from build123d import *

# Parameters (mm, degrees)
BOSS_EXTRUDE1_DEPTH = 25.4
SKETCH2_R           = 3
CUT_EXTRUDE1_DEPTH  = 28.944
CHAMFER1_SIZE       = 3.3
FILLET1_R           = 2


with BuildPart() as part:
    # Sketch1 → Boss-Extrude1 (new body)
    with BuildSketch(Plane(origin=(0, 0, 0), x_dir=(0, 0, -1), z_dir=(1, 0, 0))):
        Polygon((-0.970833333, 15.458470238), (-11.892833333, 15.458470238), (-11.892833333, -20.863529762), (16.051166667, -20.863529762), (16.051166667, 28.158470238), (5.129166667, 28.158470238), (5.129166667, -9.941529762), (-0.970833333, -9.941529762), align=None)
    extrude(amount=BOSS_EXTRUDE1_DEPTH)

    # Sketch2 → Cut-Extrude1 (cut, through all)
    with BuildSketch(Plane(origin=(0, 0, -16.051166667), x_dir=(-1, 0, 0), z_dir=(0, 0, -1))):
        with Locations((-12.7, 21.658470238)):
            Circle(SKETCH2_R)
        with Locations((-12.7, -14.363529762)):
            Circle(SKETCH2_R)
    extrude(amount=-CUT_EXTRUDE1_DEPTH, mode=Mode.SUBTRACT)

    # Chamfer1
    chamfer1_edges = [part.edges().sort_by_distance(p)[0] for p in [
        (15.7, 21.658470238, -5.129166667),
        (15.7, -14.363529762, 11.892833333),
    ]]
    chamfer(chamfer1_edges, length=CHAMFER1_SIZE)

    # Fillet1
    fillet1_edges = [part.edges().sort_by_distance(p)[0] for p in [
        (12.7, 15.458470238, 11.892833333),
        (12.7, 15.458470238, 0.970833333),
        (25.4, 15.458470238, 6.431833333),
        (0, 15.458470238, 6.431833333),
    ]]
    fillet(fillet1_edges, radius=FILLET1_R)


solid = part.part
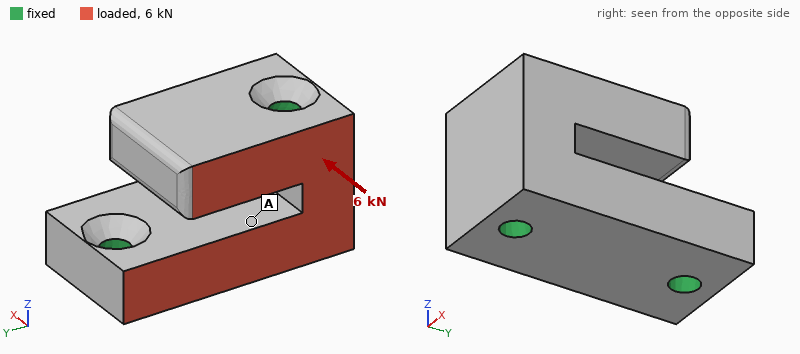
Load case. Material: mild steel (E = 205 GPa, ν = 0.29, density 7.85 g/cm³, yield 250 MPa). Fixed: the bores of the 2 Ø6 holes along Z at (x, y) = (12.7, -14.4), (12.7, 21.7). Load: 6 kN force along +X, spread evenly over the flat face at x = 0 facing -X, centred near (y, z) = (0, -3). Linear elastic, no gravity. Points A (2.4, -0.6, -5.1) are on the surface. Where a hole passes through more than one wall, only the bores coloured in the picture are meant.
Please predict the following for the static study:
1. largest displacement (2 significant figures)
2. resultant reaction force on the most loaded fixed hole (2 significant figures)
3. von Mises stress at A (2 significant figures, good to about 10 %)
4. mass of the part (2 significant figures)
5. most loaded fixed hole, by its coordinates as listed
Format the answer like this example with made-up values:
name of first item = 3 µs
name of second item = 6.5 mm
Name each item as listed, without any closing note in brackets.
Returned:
largest displacement = 8.3 µm
resultant reaction force on the most loaded fixed hole = 4.3 kN
von Mises stress at A = 7.4 MPa
mass of the part = 190 g
most loaded fixed hole, by its coordinates as listed = (12.7, -14.4)
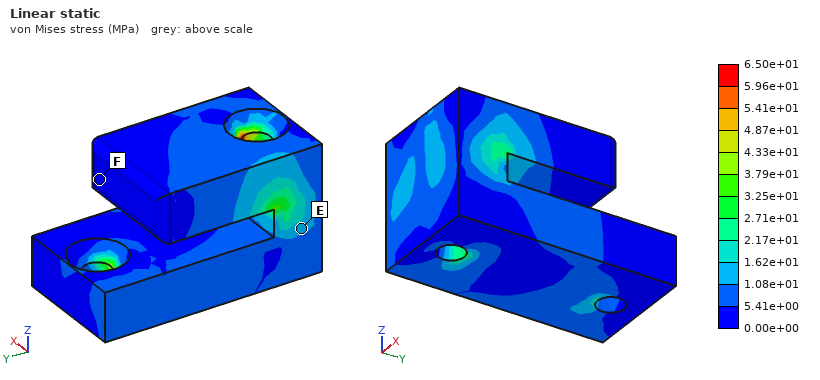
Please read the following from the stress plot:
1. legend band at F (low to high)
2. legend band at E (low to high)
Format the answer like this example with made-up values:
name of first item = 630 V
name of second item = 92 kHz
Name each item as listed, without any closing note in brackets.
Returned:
legend band at F = 0.00e+00 to 5.41e+00 MPa
legend band at E = 1.08e+01 to 1.62e+01 MPa
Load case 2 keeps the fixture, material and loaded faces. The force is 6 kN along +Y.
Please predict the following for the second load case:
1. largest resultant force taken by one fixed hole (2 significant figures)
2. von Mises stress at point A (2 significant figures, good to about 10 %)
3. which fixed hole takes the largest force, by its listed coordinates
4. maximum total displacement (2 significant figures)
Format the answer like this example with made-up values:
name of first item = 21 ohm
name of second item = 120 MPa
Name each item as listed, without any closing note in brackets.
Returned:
largest resultant force taken by one fixed hole = 4.6 kN
von Mises stress at point A = 13 MPa
which fixed hole takes the largest force, by its listed coordinates = (12.7, -14.4)
maximum total displacement = 10 µm
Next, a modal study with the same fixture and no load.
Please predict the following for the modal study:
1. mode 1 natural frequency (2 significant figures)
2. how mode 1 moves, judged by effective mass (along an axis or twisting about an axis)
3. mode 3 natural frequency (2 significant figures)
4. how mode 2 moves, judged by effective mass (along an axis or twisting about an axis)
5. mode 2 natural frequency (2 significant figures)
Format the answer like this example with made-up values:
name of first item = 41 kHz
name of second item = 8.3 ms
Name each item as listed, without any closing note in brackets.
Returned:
mode 1 natural frequency = 8700 Hz
how mode 1 moves, judged by effective mass = along Z
mode 3 natural frequency = 19 kHz
how mode 2 moves, judged by effective mass = along X
mode 2 natural frequency = 11 kHz
